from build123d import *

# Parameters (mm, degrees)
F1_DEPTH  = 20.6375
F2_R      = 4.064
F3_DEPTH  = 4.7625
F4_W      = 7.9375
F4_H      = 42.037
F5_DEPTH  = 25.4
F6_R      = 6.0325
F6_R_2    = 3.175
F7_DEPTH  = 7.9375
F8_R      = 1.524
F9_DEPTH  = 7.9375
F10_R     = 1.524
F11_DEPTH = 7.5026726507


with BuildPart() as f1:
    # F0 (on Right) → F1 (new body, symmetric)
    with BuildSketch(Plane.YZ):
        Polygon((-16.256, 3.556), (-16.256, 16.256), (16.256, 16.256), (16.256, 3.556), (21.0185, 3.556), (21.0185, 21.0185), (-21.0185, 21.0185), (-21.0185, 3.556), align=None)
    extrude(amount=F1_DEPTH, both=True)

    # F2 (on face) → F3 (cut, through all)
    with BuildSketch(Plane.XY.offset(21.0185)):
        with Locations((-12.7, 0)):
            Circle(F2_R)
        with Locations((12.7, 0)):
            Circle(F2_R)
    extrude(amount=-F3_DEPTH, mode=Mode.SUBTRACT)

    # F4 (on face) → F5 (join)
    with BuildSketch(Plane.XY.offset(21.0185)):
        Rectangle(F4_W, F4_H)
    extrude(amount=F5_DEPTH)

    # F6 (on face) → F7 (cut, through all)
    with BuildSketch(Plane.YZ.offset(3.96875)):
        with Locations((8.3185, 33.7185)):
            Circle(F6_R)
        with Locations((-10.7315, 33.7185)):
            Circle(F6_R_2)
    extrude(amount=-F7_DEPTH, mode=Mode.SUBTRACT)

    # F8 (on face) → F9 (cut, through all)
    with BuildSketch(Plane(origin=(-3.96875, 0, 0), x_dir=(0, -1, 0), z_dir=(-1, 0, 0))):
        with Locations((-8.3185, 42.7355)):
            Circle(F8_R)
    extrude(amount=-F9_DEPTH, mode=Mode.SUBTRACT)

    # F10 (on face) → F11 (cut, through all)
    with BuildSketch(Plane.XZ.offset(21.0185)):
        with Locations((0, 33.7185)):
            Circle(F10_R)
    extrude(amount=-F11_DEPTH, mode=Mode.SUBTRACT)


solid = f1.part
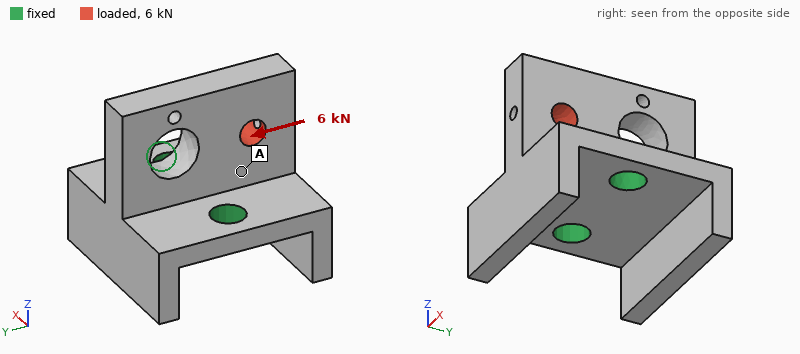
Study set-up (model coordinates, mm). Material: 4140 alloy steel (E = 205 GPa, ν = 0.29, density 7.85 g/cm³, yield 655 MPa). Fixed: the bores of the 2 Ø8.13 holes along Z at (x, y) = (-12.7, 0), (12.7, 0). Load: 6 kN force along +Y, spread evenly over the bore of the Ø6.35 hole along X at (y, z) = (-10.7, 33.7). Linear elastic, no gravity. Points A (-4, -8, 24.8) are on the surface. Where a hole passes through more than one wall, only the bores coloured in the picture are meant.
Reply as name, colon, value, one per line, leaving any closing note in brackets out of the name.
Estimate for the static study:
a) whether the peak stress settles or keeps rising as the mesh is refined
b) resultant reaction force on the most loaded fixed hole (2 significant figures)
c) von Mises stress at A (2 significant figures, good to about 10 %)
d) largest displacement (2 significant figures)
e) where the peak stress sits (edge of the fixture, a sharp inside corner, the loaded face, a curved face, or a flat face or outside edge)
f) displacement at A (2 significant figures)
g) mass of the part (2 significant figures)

whether the peak stress settles or keeps rising as the mesh is refined: keeps rising
resultant reaction force on the most loaded fixed hole: 3.0 kN
von Mises stress at A: 63 MPa
largest displacement: 81 µm
where the peak stress sits: edge of the fixture
displacement at A: 23 µm
mass of the part: 160 g
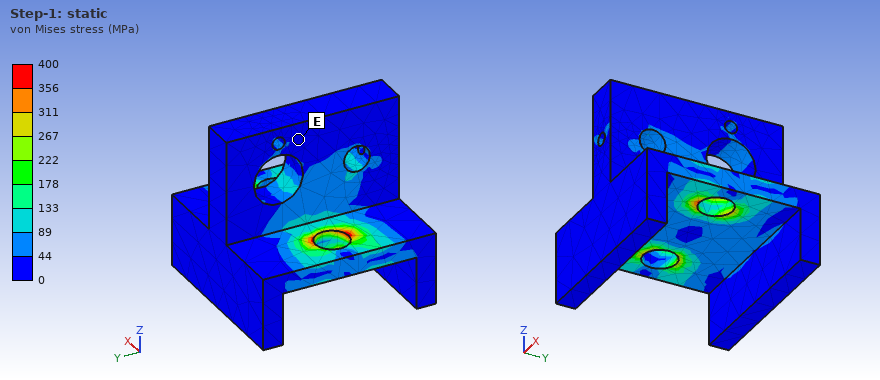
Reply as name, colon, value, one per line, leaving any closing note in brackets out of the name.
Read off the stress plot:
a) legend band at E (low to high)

legend band at E: 0 to 44 MPa
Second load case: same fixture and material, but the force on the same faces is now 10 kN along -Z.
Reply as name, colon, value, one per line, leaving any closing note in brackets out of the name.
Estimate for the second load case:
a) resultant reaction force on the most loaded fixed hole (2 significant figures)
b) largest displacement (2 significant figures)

resultant reaction force on the most loaded fixed hole: 5.2 kN
largest displacement: 96 µm
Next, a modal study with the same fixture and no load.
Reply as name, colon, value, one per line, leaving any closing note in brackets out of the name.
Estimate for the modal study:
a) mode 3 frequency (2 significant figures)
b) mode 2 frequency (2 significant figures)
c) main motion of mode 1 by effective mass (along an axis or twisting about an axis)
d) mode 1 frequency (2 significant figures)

mode 3 frequency: 9100 Hz
mode 2 frequency: 6500 Hz
main motion of mode 1 by effective mass: twisting about X
mode 1 frequency: 4500 Hz
